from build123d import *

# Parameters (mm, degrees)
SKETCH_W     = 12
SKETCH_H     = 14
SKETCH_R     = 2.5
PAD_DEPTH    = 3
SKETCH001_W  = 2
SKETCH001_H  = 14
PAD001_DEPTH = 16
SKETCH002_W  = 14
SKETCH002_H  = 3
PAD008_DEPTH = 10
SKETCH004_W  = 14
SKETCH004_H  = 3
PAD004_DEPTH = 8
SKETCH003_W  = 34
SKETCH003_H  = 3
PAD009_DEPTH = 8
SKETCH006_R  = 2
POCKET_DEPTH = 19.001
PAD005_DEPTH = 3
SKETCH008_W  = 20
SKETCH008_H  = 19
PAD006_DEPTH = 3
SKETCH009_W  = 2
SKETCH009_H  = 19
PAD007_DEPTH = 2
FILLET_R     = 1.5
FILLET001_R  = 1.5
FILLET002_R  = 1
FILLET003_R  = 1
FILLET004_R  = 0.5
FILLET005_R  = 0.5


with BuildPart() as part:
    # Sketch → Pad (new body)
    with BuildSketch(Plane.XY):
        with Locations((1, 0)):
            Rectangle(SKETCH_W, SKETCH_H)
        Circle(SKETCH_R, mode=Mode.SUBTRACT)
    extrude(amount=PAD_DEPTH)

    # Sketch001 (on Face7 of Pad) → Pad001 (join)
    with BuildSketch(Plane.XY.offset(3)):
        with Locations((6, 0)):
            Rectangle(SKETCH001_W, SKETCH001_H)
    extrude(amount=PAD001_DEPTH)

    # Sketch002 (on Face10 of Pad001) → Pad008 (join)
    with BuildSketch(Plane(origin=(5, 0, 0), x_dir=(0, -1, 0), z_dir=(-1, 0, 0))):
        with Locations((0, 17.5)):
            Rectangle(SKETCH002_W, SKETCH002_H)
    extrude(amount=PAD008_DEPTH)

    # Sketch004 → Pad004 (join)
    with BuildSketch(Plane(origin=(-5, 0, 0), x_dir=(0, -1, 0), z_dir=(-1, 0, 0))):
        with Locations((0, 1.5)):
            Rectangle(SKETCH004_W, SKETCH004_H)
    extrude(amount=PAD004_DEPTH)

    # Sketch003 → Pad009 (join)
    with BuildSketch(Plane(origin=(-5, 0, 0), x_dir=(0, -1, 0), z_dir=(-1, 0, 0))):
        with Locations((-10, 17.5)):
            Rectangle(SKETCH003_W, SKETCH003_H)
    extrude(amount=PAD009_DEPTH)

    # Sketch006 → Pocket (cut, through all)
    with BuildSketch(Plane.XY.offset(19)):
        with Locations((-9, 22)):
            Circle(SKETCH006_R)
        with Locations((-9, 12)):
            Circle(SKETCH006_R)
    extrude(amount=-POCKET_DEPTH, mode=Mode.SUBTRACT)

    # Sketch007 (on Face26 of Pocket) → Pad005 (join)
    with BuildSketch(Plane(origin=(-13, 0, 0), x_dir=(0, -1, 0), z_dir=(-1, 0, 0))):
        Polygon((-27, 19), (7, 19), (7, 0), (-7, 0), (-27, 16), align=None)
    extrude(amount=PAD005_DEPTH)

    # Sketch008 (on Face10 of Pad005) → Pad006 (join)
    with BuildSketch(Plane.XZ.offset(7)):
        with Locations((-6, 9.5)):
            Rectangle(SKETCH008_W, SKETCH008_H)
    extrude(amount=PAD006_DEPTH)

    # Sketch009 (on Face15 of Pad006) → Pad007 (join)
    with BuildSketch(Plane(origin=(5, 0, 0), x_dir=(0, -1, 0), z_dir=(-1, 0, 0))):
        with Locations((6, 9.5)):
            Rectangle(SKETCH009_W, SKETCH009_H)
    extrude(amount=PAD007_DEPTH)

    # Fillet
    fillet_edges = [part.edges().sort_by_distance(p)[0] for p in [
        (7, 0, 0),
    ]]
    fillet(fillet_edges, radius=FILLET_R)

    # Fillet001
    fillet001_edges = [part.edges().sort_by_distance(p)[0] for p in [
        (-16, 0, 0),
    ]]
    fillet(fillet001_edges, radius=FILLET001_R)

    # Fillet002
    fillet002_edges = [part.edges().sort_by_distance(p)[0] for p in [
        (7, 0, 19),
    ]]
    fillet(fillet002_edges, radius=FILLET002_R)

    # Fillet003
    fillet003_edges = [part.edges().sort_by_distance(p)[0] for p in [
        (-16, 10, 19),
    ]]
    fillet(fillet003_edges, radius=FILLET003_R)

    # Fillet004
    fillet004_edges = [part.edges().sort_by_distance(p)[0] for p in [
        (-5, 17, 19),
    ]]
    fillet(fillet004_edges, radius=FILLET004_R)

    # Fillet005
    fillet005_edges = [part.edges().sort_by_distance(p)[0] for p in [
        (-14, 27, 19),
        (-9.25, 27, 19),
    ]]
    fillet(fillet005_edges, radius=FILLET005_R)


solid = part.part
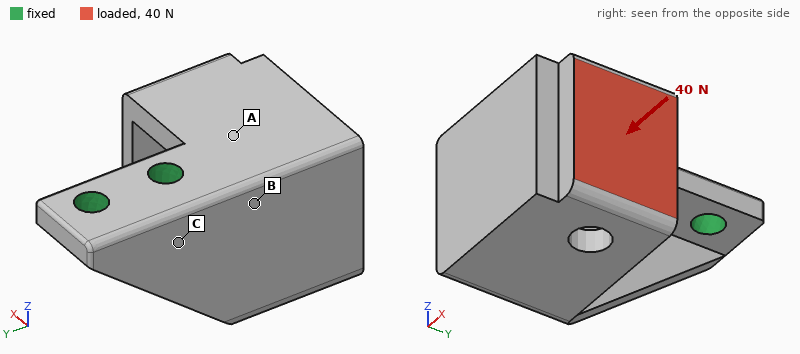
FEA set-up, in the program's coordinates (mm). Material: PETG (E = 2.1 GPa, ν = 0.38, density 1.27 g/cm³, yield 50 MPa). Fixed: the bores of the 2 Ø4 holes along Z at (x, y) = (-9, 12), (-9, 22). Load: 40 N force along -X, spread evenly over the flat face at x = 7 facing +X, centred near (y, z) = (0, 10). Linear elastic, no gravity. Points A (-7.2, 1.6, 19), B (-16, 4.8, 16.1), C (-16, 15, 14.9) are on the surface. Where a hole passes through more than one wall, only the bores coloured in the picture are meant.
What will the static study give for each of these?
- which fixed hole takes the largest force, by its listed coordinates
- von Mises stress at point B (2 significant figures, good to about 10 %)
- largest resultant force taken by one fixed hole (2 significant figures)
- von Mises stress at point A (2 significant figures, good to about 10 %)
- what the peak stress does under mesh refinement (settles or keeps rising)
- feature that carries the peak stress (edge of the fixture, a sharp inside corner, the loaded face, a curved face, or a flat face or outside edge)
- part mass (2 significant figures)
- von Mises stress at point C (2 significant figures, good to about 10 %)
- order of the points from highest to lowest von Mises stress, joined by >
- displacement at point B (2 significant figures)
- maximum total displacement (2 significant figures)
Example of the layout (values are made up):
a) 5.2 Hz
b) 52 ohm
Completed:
a) (-9, 12)
b) 3.9 MPa
c) 62 N
d) 1.8 MPa
e) keeps rising
f) edge of the fixture
g) 6.4 g
h) 6.0 MPa
i) C > B > A
j) 0.10 mm
k) 0.54 mm
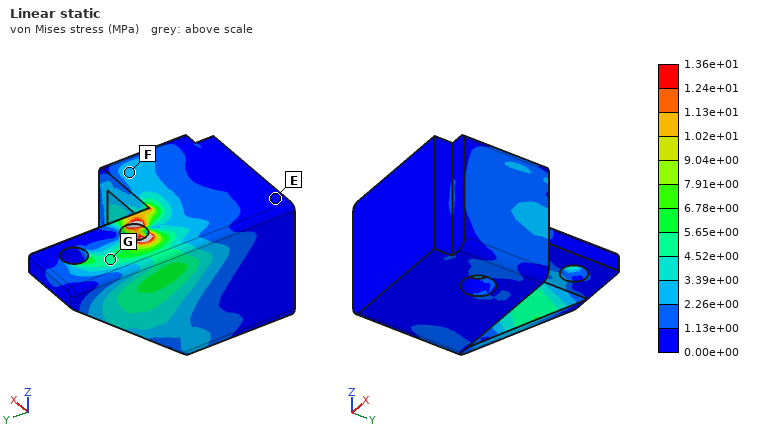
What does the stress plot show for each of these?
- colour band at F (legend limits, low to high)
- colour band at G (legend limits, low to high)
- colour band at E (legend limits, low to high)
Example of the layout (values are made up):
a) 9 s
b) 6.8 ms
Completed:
a) 2.26e+00 to 3.39e+00 MPa
b) 4.52e+00 to 5.65e+00 MPa
c) 0.00e+00 to 1.13e+00 MPa
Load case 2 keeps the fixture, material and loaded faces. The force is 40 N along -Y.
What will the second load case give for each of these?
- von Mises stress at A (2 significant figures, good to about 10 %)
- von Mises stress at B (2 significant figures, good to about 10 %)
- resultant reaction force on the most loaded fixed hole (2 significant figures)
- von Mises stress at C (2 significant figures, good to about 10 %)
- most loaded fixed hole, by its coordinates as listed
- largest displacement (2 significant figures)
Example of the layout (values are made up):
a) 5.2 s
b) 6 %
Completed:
a) 2.8 MPa
b) 5.7 MPa
c) 69 N
d) 4.1 MPa
e) (-9, 12)
f) 0.49 mm
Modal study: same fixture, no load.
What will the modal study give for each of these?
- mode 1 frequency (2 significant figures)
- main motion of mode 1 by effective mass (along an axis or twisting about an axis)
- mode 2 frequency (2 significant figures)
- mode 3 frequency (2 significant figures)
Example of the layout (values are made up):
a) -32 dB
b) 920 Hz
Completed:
a) 630 Hz
b) along X
c) 910 Hz
d) 1700 Hz
